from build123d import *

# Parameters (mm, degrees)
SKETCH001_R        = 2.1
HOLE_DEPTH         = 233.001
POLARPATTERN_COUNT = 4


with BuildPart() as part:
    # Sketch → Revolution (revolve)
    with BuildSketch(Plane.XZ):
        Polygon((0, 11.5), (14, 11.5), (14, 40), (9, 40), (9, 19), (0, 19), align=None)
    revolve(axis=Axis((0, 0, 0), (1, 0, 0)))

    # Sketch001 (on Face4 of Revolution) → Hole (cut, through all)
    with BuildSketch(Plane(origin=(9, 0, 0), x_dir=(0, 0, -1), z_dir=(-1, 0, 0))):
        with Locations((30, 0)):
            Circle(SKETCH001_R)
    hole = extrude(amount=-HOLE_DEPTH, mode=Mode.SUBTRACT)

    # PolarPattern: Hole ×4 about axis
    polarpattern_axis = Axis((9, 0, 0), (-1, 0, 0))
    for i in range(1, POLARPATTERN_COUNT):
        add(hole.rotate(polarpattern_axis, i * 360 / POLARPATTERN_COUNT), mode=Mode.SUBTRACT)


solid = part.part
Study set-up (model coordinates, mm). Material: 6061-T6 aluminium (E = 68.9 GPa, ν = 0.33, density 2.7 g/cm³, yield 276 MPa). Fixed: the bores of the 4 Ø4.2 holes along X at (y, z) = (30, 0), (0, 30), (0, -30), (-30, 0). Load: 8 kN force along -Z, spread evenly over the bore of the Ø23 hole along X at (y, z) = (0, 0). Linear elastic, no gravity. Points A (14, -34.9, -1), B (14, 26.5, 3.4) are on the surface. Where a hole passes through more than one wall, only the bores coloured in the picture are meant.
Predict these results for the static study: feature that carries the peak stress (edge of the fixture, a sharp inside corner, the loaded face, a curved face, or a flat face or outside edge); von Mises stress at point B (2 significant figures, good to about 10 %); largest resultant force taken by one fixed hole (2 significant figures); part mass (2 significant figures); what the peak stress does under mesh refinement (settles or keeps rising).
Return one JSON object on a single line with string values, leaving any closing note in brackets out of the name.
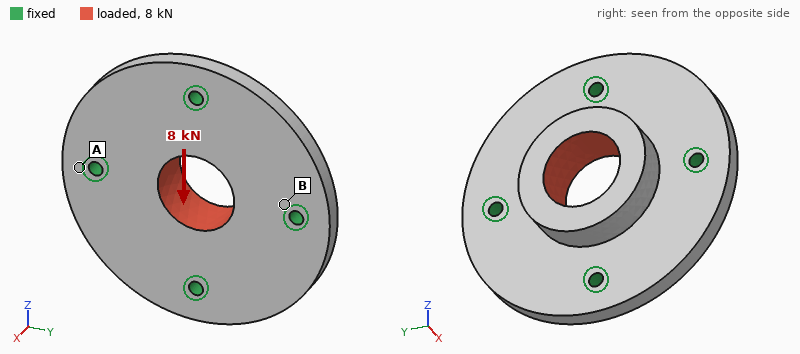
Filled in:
{"feature that carries the peak stress": "edge of the fixture", "von Mises stress at point B": "13 MPa", "largest resultant force taken by one fixed hole": "2.5 kN", "part mass": "79 g", "what the peak stress does under mesh refinement": "keeps rising"}
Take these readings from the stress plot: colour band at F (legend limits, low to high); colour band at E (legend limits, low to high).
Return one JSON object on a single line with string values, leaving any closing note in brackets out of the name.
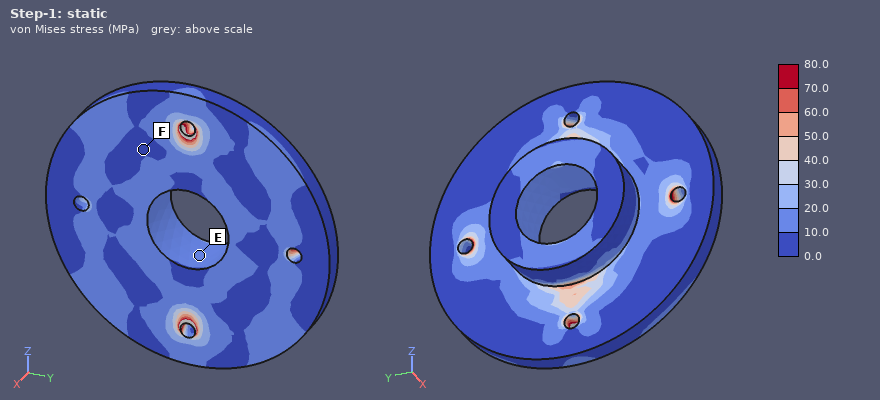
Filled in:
{"colour band at F": "0.0 to 10.0 MPa", "colour band at E": "10.0 to 20.0 MPa"}
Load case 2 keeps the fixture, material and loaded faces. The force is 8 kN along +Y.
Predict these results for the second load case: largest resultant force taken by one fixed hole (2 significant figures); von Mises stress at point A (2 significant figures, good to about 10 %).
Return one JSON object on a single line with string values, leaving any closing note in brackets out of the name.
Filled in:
{"largest resultant force taken by one fixed hole": "2.5 kN", "von Mises stress at point A": "17 MPa"}
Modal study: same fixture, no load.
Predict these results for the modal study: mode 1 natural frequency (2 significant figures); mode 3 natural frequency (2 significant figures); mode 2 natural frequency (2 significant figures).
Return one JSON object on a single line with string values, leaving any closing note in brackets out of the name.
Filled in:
{"mode 1 natural frequency": "9300 Hz", "mode 3 natural frequency": "9700 Hz", "mode 2 natural frequency": "9700 Hz"}
